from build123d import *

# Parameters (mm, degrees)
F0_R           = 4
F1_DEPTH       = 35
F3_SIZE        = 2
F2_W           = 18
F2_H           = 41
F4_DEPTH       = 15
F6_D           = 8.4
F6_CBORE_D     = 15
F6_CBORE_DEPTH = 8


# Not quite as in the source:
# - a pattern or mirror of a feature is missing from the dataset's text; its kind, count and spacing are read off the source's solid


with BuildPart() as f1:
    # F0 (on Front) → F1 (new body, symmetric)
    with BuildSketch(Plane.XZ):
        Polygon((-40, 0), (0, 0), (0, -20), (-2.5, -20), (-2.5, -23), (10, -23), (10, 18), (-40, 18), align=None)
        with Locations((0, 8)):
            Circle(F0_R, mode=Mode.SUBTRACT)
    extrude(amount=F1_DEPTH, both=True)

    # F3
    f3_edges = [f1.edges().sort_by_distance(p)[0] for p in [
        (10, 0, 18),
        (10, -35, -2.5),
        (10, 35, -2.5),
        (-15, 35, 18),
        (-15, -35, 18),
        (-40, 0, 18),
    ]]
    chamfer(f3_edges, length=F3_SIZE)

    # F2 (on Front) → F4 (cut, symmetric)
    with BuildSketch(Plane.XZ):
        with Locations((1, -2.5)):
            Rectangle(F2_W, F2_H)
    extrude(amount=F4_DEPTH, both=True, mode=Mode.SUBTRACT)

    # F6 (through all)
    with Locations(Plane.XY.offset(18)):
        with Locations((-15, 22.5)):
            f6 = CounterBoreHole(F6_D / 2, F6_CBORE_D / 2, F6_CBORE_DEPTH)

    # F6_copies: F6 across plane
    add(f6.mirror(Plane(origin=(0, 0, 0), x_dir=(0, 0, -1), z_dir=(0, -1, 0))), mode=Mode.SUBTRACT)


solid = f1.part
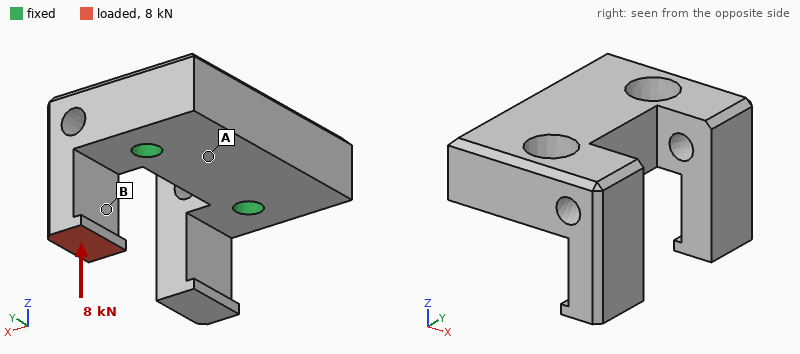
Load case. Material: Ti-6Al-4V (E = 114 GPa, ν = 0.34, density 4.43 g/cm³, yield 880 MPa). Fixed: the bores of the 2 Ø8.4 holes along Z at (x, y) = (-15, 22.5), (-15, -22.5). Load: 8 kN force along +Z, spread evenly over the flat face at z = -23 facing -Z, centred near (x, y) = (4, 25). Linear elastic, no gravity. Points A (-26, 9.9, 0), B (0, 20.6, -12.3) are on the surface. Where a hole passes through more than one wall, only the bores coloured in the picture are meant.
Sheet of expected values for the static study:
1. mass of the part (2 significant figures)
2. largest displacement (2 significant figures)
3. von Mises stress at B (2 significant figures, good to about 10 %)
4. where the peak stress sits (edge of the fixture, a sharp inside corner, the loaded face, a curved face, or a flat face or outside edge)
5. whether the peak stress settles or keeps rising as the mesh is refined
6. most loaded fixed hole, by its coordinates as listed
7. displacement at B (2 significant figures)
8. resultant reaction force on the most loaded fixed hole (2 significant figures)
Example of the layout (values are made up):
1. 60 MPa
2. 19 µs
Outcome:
1. 250 g
2. 0.12 mm
3. 72 MPa
4. edge of the fixture
5. keeps rising
6. (-15, 22.5)
7. 0.076 mm
8. 8.3 kN
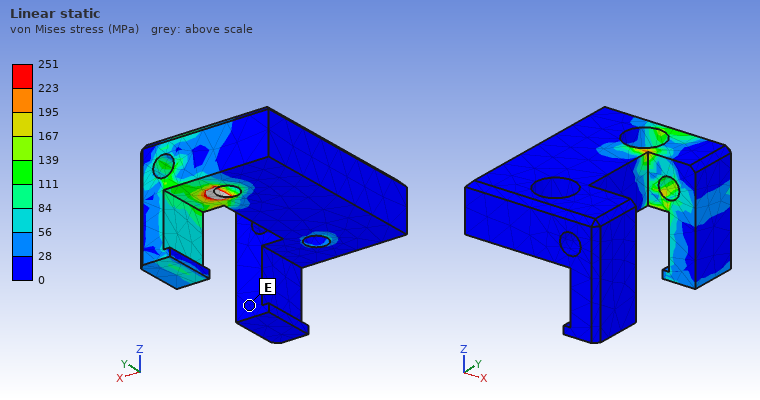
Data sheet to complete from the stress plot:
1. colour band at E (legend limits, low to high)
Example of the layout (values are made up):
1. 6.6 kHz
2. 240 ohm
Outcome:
1. 0 to 28 MPa
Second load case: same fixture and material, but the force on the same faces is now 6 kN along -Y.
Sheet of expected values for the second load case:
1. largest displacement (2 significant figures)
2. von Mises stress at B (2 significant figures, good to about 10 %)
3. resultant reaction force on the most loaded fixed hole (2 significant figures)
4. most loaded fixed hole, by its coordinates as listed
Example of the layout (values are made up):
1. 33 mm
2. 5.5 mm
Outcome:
1. 0.33 mm
2. 100 MPa
3. 8.1 kN
4. (-15, 22.5)
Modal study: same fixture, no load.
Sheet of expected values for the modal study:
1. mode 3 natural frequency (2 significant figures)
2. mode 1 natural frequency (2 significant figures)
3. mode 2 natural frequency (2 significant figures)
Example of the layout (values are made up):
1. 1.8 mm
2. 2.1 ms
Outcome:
1. 6700 Hz
2. 5600 Hz
3. 5900 Hz
